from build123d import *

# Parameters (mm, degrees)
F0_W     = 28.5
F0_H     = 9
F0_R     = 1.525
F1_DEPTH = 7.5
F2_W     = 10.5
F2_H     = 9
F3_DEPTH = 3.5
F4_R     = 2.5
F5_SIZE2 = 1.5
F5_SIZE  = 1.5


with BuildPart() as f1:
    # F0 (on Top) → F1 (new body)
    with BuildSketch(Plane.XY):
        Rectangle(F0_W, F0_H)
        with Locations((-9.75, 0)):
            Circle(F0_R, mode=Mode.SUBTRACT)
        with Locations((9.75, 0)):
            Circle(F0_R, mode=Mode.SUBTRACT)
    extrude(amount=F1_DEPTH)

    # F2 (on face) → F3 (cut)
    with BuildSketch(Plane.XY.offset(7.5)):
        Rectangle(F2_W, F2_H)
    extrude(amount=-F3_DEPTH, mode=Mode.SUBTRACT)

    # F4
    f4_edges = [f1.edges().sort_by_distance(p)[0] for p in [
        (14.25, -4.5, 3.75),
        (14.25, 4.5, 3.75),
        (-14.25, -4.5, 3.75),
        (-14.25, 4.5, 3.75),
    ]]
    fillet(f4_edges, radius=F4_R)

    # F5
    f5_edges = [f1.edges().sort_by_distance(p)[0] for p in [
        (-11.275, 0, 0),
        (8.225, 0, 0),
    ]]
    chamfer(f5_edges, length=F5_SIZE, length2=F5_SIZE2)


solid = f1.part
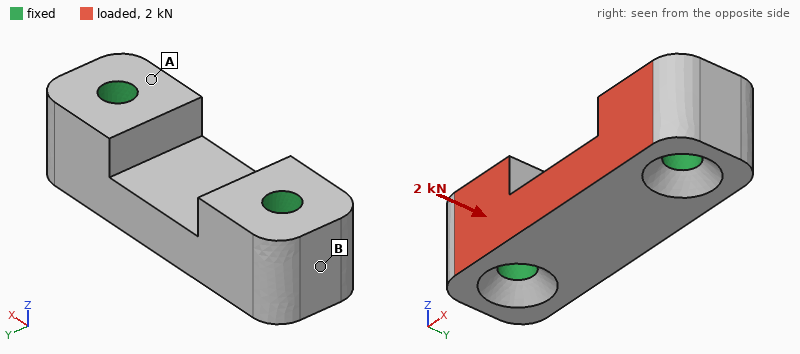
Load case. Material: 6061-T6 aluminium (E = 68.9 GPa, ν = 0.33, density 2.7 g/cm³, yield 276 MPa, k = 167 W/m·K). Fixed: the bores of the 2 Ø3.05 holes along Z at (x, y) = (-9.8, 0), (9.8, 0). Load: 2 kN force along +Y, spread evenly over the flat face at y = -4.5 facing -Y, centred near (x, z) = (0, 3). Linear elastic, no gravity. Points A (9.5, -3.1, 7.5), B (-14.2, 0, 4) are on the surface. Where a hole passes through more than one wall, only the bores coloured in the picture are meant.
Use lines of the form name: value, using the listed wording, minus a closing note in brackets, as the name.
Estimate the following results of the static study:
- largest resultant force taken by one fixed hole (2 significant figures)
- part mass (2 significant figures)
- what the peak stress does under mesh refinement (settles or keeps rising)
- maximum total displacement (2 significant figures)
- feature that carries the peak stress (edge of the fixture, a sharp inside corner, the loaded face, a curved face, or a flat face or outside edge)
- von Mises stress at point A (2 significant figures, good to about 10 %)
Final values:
largest resultant force taken by one fixed hole: 1.0 kN
part mass: 3.8 g
what the peak stress does under mesh refinement: keeps rising
maximum total displacement: 6.6 µm
feature that carries the peak stress: edge of the fixture
von Mises stress at point A: 20 MPa
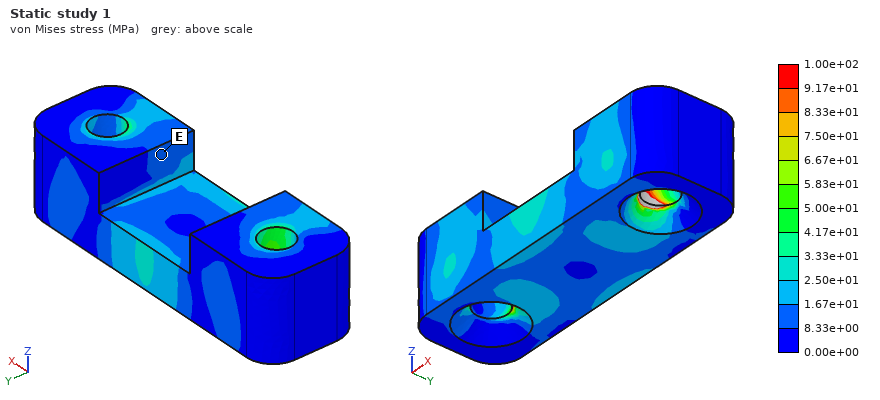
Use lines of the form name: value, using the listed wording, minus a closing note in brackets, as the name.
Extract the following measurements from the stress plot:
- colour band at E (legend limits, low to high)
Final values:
colour band at E: 8.33e+00 to 1.67e+01 MPa
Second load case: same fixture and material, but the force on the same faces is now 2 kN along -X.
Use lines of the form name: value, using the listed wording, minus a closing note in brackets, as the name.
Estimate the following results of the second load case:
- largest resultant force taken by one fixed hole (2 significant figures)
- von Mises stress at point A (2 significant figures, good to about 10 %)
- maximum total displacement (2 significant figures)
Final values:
largest resultant force taken by one fixed hole: 1.0 kN
von Mises stress at point A: 24 MPa
maximum total displacement: 4.7 µm
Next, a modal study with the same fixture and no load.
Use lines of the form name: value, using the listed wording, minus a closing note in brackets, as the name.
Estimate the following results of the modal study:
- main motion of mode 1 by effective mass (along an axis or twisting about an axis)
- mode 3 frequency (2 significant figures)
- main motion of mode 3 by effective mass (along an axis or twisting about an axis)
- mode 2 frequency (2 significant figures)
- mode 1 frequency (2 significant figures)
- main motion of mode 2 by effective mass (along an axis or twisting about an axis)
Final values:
main motion of mode 1 by effective mass: along Y
mode 3 frequency: 79 kHz
main motion of mode 3 by effective mass: twisting about X
mode 2 frequency: 61 kHz
mode 1 frequency: 58 kHz
main motion of mode 2 by effective mass: along Z
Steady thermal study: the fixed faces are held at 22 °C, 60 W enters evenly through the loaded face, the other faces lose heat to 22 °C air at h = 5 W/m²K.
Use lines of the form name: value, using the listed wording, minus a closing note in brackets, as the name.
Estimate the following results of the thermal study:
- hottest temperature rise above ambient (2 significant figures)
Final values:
hottest temperature rise above ambient: 20 K
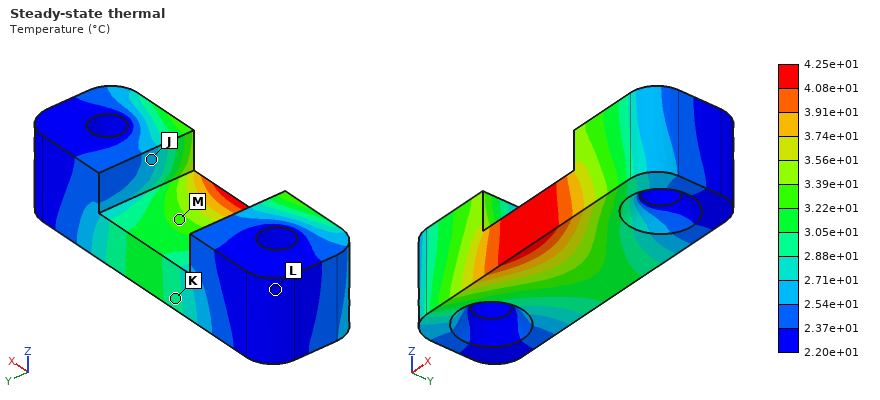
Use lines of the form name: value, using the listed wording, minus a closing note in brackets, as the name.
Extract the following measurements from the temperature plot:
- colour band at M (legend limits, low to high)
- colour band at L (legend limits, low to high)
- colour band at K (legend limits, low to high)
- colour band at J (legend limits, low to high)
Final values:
colour band at M: 3.22e+01 to 3.39e+01 °C
colour band at L: 2.20e+01 to 2.37e+01 °C
colour band at K: 2.88e+01 to 3.05e+01 °C
colour band at J: 2.54e+01 to 2.71e+01 °C
